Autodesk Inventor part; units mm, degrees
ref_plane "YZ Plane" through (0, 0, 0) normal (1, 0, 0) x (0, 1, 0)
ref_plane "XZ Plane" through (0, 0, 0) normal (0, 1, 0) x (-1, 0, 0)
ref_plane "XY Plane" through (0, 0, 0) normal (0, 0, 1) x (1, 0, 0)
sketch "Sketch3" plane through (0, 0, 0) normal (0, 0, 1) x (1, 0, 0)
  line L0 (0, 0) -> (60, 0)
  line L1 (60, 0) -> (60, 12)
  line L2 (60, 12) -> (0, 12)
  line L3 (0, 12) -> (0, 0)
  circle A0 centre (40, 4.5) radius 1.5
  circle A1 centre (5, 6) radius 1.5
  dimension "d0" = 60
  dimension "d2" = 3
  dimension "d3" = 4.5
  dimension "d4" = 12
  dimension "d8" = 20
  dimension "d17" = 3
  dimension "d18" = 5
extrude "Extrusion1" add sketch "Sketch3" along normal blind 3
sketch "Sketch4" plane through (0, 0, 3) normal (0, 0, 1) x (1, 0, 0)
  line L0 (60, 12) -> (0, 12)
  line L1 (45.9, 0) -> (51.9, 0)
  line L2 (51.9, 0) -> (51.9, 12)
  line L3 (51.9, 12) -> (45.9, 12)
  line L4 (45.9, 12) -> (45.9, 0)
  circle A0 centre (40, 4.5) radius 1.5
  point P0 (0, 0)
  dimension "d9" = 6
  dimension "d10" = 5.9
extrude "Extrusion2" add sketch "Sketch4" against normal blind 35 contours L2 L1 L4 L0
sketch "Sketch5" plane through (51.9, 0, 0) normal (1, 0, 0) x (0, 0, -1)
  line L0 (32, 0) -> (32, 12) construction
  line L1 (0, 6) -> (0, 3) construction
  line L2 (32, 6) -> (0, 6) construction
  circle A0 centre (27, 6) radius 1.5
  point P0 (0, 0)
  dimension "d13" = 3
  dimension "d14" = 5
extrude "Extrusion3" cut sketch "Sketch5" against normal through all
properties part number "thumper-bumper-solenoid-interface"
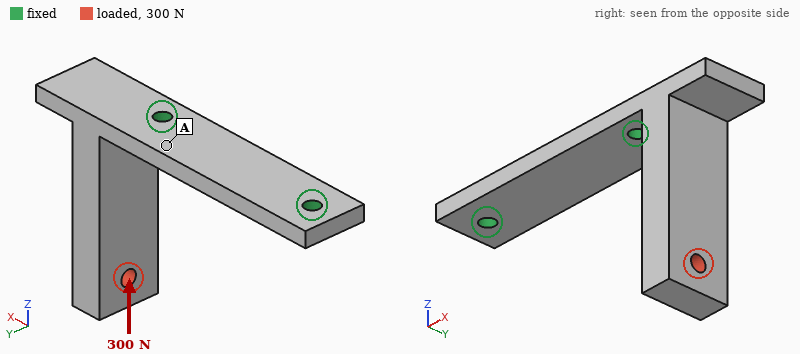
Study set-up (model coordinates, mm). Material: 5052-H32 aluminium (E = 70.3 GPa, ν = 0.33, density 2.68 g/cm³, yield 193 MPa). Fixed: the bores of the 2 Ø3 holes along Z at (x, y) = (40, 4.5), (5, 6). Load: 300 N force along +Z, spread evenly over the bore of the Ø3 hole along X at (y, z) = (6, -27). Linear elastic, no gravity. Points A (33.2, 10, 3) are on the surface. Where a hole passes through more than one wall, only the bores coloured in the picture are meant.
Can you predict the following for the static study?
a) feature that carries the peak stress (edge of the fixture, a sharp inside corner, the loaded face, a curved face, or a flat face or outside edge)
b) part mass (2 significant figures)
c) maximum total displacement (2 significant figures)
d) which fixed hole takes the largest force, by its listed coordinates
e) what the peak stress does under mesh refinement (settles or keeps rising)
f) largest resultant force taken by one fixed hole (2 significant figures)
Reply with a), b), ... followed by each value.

a) edge of the fixture
b) 12 g
c) 0.20 mm
d) (40, 4.5)
e) keeps rising
f) 310 N
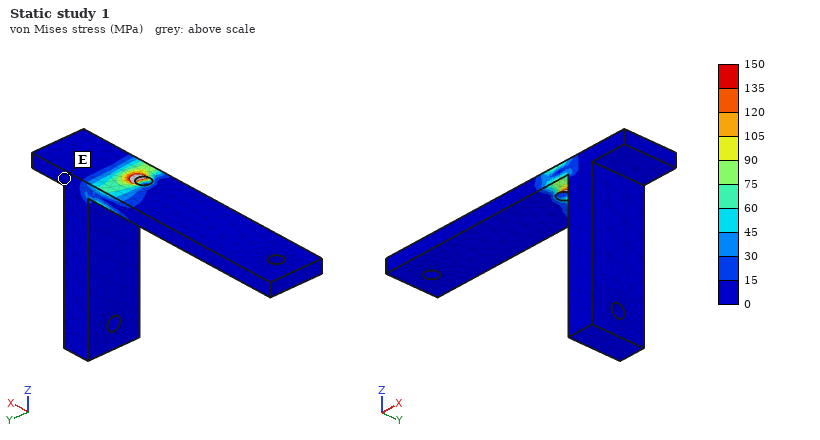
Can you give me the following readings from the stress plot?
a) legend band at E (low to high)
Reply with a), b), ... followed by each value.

a) 0 to 15 MPa
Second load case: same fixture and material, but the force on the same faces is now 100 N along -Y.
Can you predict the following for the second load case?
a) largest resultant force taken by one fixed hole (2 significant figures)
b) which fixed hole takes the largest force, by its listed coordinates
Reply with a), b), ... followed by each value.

a) 120 N
b) (40, 4.5)
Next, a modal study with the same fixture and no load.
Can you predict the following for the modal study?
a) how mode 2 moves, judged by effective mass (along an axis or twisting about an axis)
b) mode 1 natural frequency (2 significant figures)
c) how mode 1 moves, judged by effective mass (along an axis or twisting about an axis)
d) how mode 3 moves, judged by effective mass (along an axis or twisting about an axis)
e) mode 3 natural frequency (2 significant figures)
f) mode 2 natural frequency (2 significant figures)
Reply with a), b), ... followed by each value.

a) along Y
b) 1500 Hz
c) along X
d) along Z
e) 9300 Hz
f) 2200 Hz
